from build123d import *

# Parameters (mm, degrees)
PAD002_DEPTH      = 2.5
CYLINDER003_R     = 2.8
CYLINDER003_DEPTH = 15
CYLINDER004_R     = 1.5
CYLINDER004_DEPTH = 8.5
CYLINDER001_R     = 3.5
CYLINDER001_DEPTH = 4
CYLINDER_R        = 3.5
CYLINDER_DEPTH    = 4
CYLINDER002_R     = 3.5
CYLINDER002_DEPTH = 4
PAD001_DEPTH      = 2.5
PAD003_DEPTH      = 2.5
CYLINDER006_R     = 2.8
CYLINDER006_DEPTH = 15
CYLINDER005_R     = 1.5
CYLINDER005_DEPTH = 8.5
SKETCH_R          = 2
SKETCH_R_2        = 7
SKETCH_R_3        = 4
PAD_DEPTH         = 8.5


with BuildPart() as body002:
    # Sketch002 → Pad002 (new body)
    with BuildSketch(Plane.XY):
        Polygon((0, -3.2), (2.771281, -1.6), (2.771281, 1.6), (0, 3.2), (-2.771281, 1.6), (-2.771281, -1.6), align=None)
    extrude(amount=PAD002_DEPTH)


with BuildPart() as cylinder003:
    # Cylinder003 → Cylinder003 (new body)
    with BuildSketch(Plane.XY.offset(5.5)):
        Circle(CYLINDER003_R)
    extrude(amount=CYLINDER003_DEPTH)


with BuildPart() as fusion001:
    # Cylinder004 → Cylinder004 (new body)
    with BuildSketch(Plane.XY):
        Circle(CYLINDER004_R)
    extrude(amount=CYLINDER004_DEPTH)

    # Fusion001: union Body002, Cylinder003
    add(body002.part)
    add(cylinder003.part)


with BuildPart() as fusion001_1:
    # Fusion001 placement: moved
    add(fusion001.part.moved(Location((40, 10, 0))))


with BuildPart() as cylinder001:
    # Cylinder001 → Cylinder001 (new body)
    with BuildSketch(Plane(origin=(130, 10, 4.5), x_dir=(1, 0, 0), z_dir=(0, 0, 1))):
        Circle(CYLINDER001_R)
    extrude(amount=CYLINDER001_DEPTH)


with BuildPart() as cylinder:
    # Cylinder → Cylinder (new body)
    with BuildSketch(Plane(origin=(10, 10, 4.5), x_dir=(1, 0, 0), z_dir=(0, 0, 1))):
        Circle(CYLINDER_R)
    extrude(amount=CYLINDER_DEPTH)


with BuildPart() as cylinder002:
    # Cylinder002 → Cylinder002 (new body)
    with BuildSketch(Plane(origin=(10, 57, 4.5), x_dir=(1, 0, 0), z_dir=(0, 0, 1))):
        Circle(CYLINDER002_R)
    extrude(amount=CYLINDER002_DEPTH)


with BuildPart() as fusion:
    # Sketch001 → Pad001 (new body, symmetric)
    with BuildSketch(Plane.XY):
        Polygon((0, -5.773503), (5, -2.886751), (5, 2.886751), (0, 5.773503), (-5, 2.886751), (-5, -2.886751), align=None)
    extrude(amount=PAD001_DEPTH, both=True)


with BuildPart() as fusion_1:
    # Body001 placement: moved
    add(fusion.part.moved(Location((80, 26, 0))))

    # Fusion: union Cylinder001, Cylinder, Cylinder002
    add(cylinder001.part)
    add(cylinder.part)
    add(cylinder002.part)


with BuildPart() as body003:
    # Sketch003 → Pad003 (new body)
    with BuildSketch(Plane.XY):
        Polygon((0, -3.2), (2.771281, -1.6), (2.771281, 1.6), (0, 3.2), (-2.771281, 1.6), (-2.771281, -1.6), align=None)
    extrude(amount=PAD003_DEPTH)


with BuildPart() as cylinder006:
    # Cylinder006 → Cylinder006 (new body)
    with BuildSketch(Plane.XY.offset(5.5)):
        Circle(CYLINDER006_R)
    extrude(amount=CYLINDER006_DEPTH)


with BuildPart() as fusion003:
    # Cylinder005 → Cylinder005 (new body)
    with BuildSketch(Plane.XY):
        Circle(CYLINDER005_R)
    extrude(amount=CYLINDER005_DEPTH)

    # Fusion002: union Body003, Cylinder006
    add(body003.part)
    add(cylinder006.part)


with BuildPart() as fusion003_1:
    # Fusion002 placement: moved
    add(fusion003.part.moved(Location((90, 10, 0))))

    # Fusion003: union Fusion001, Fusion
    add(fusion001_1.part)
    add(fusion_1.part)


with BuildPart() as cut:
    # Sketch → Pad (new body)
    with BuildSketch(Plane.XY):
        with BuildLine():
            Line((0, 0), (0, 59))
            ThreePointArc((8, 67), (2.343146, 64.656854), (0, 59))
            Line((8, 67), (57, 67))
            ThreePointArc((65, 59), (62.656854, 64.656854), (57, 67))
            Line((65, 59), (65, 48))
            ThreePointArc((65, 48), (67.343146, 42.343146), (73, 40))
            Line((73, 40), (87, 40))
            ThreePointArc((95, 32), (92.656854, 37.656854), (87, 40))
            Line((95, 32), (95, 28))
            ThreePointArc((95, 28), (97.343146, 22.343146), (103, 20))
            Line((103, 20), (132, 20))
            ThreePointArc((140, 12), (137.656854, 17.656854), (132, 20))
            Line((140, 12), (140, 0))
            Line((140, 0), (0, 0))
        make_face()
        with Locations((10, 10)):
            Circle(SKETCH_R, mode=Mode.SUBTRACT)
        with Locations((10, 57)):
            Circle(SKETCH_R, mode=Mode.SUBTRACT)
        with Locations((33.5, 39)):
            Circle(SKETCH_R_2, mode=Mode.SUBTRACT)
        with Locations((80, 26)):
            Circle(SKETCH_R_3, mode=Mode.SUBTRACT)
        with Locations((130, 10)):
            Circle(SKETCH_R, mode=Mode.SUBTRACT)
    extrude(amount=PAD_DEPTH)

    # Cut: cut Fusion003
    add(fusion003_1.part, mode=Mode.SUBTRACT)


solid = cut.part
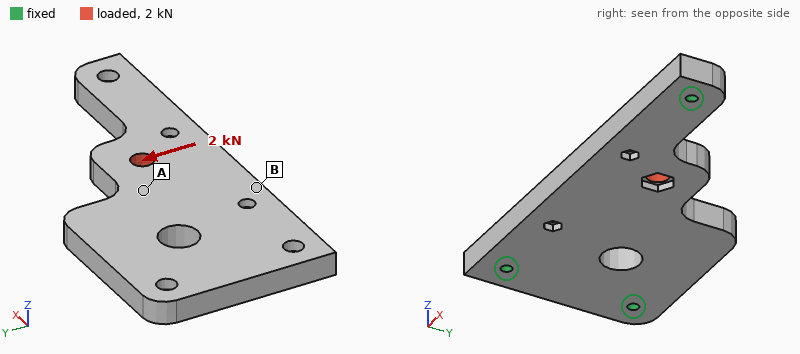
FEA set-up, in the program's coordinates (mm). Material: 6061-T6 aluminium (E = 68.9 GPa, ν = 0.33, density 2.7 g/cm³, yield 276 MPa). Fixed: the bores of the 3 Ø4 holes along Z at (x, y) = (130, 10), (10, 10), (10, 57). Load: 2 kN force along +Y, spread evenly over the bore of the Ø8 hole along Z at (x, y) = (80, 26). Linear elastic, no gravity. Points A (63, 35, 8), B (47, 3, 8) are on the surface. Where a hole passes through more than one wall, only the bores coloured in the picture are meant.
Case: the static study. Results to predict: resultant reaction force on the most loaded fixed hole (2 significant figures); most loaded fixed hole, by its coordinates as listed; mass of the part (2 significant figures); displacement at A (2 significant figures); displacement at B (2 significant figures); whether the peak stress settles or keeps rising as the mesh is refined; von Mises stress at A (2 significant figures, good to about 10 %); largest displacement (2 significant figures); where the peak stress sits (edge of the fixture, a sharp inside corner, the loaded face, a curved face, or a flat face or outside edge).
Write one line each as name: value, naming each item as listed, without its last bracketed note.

resultant reaction force on the most loaded fixed hole: 1.8 kN
most loaded fixed hole, by its coordinates as listed: (10, 57)
mass of the part: 140 g
displacement at A: 18 µm
displacement at B: 14 µm
whether the peak stress settles or keeps rising as the mesh is refined: keeps rising
von Mises stress at A: 12 MPa
largest displacement: 28 µm
where the peak stress sits: edge of the fixture
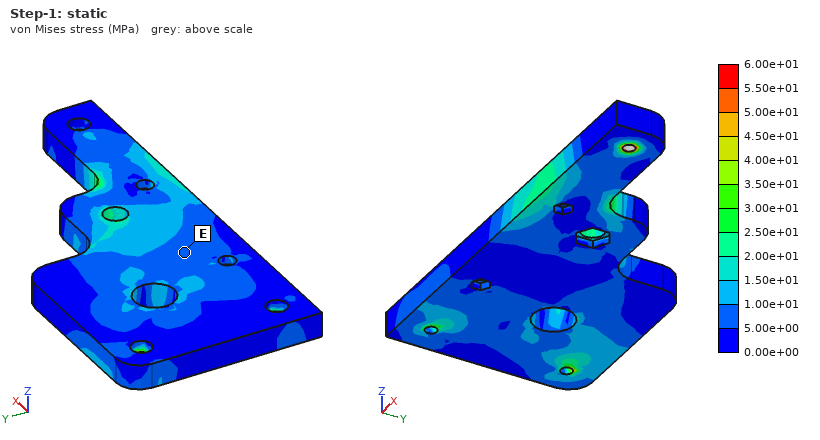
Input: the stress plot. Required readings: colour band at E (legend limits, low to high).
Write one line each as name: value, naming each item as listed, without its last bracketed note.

colour band at E: 5.00e+00 to 1.00e+01 MPa
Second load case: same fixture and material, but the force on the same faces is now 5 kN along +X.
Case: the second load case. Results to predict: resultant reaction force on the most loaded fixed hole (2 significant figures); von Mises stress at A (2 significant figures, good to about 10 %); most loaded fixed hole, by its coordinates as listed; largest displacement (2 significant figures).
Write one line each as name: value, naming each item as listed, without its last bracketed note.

resultant reaction force on the most loaded fixed hole: 2.2 kN
von Mises stress at A: 17 MPa
most loaded fixed hole, by its coordinates as listed: (10, 10)
largest displacement: 21 µm
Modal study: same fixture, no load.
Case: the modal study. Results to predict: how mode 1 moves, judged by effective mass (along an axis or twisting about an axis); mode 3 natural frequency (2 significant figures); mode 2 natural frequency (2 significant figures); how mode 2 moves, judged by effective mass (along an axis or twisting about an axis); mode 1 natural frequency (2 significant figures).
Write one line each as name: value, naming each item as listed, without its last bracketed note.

how mode 1 moves, judged by effective mass: along Z
mode 3 natural frequency: 5900 Hz
mode 2 natural frequency: 3700 Hz
how mode 2 moves, judged by effective mass: twisting about X
mode 1 natural frequency: 1900 Hz
